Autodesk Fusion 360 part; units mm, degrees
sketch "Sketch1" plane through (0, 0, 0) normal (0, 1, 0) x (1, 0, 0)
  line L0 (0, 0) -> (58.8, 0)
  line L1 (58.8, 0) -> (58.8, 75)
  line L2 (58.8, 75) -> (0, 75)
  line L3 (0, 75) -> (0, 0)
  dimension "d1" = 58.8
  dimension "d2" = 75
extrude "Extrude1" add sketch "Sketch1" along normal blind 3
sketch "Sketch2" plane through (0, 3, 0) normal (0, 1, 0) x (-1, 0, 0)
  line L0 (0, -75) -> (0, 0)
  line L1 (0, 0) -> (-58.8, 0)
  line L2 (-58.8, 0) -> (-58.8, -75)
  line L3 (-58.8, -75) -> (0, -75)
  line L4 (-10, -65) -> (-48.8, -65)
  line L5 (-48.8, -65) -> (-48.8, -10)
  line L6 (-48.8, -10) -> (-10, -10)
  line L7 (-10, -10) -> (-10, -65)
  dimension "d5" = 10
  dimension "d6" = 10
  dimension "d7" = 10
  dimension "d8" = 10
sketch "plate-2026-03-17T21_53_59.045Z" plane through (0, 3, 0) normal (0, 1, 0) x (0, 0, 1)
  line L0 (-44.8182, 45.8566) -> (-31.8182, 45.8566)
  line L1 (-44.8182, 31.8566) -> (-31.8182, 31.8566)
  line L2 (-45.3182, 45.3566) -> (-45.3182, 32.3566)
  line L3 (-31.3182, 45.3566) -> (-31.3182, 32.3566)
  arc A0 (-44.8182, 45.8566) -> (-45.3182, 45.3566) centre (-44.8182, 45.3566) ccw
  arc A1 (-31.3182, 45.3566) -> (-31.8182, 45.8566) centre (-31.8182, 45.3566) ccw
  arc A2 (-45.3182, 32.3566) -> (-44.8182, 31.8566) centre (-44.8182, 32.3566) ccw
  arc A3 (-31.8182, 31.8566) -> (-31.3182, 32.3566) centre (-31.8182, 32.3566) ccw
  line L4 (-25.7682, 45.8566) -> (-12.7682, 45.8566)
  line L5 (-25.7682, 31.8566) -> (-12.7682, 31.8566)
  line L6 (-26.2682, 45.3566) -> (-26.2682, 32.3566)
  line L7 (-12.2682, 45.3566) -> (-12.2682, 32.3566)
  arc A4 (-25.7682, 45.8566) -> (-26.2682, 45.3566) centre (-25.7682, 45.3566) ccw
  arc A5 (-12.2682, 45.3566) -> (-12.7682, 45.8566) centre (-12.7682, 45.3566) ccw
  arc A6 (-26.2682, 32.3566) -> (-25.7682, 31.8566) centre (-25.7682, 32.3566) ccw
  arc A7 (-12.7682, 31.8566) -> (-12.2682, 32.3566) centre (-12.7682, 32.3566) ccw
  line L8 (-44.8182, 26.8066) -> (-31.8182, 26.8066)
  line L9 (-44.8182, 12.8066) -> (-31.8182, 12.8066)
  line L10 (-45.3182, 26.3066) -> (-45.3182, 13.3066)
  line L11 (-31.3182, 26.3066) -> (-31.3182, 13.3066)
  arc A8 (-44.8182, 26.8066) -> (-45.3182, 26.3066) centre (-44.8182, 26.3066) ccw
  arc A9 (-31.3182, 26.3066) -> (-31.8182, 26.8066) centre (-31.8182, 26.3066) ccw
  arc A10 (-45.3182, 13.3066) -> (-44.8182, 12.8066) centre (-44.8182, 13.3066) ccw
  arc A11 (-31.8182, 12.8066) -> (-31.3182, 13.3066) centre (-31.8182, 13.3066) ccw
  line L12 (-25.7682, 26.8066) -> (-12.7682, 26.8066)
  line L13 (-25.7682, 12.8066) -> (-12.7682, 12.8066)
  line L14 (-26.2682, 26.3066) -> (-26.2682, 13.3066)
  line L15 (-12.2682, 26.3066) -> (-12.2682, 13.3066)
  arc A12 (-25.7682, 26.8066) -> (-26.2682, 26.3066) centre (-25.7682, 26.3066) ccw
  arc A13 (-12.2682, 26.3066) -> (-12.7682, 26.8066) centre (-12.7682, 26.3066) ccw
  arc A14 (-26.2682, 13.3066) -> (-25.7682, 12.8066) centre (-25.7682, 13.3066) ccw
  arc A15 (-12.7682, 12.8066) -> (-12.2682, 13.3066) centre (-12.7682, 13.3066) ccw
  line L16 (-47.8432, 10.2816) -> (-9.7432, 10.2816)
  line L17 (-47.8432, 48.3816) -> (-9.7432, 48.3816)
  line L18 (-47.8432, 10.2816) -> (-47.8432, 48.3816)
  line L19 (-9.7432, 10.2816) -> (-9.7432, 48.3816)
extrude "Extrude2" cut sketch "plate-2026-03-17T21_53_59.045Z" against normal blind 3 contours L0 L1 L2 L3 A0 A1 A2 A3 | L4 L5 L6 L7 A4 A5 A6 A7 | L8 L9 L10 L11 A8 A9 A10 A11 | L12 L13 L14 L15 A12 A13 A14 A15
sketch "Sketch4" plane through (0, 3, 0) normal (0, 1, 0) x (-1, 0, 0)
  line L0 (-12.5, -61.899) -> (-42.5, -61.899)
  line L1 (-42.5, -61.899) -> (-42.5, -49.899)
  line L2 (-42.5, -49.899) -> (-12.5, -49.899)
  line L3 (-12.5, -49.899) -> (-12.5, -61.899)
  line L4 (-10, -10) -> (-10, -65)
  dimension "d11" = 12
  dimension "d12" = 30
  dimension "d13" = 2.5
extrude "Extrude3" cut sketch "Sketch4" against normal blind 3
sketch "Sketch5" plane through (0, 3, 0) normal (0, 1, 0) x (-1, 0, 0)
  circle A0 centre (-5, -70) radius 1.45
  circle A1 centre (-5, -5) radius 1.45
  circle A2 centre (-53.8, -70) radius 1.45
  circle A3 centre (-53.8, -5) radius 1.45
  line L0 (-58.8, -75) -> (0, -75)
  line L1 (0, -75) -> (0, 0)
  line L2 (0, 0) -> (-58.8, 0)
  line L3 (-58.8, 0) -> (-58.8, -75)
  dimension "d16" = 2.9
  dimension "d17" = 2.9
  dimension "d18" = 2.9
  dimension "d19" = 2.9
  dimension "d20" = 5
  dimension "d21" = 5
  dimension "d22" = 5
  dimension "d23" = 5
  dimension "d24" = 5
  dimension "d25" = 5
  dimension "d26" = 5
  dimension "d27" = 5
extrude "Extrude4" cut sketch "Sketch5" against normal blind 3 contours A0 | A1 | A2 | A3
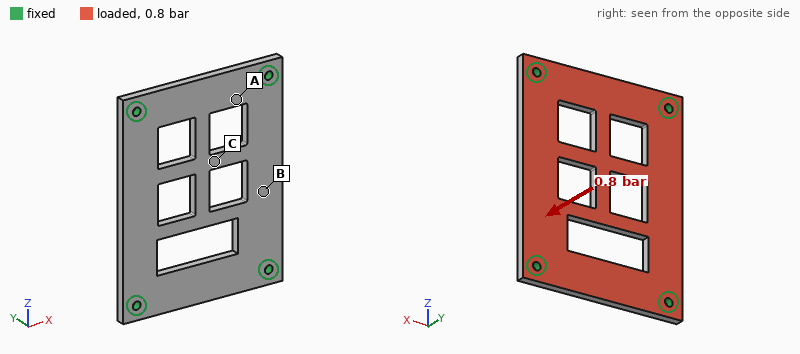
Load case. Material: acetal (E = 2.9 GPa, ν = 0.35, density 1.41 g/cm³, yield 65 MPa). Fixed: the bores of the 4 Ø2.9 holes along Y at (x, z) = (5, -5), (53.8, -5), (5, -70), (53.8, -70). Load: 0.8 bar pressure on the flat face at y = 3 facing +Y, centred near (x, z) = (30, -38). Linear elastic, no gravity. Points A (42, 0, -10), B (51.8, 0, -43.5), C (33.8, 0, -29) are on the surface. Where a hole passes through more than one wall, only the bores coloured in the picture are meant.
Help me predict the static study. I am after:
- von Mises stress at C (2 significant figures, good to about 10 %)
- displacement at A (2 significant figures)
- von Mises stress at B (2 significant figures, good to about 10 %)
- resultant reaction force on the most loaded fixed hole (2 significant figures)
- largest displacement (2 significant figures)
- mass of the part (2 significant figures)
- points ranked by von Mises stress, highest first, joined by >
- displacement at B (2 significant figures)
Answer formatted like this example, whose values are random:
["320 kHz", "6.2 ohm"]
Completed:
["6.7 MPa", "0.23 mm", "10 MPa", "67 N", "1.0 mm", "14 g", "B > C > A", "0.69 mm"]
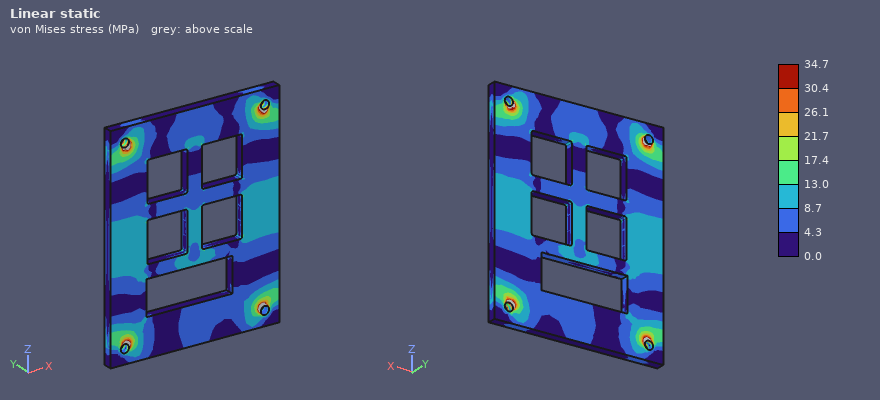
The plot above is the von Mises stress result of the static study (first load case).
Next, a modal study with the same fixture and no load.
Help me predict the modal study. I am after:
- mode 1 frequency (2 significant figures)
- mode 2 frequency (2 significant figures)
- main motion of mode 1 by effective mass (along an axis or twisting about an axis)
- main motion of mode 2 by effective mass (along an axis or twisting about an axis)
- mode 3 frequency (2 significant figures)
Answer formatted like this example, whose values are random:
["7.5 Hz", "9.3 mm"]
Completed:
["860 Hz", "1200 Hz", "along Y", "twisting about Z", "1600 Hz"]
